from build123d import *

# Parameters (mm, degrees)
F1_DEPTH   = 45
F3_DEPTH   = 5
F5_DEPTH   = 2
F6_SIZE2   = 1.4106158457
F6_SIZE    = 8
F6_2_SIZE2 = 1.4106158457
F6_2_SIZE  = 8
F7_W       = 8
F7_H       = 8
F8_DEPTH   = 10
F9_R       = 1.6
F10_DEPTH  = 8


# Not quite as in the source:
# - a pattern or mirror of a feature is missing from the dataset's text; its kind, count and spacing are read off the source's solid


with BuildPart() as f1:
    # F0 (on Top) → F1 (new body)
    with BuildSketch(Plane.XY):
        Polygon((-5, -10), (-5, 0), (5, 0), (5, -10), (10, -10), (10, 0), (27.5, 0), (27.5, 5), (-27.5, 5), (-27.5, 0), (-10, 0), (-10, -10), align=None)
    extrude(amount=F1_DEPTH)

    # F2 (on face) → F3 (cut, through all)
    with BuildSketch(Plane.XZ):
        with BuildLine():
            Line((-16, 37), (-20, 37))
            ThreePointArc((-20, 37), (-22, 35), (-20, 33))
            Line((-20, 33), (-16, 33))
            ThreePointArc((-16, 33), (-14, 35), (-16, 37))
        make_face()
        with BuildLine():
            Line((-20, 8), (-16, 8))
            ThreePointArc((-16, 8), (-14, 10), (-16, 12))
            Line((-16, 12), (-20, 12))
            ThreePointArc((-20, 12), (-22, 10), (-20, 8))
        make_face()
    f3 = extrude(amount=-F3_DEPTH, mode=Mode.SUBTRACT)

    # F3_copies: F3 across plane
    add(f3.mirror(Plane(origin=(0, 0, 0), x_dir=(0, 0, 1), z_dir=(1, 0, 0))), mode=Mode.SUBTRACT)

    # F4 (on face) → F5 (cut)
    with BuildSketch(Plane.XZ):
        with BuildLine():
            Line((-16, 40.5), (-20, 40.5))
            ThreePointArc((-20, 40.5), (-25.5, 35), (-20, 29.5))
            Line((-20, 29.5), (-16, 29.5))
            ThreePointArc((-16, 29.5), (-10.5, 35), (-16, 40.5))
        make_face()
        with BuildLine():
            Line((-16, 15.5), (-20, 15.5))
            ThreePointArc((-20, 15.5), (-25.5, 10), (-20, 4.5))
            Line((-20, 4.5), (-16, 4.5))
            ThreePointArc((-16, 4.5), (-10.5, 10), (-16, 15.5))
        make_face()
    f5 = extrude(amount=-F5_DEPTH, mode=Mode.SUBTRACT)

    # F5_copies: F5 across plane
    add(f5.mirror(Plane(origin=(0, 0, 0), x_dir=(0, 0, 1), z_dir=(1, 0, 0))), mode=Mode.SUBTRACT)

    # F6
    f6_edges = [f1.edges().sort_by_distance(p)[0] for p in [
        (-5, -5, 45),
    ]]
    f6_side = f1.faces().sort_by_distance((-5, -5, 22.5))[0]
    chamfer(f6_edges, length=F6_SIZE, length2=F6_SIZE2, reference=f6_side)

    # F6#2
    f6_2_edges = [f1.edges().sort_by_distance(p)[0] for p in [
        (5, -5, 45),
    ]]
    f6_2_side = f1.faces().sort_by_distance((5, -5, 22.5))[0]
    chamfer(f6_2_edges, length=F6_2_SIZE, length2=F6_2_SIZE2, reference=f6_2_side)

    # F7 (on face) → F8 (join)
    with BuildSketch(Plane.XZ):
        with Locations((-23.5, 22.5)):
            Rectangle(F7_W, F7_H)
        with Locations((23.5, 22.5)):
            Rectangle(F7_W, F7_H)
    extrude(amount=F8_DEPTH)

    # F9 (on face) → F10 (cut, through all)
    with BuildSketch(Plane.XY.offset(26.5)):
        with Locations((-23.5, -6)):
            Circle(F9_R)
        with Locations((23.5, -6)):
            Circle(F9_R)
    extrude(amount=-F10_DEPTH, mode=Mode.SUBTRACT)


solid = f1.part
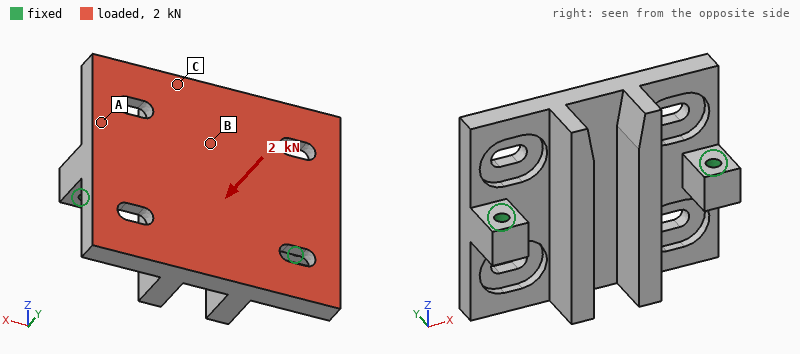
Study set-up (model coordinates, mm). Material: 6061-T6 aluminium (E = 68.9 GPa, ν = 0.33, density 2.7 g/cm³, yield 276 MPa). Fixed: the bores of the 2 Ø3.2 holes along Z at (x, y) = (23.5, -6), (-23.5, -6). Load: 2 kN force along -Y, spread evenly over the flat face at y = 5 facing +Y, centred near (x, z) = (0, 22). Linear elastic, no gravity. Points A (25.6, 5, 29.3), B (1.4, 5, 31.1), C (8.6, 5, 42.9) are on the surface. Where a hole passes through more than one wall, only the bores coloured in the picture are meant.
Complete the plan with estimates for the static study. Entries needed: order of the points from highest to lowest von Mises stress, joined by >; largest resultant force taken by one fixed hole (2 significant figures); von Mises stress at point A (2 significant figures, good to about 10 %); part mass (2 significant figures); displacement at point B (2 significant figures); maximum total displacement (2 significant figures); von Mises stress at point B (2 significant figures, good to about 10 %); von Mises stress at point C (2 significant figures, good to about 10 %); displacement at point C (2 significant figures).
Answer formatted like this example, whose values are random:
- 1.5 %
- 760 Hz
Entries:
- B > A > C
- 1.2 kN
- 20 MPa
- 44 g
- 32 µm
- 36 µm
- 27 MPa
- 5.6 MPa
- 32 µm
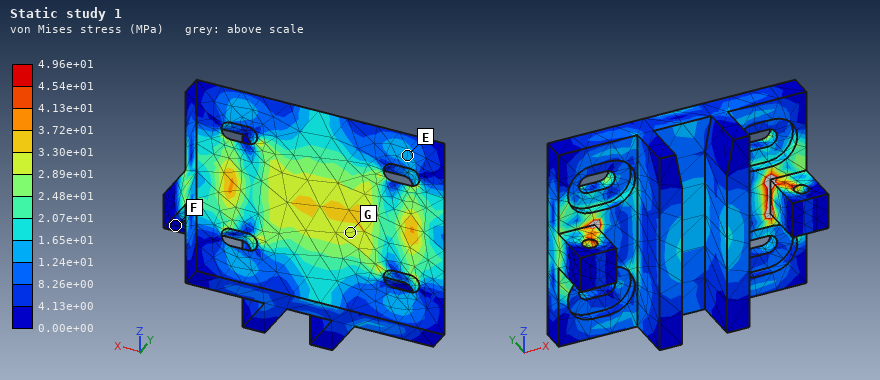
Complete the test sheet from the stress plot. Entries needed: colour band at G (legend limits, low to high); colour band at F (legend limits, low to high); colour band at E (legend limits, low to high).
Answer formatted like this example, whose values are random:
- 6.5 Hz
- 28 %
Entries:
- 2.89e+01 to 3.30e+01 MPa
- 0.00e+00 to 4.13e+00 MPa
- 1.24e+01 to 1.65e+01 MPa
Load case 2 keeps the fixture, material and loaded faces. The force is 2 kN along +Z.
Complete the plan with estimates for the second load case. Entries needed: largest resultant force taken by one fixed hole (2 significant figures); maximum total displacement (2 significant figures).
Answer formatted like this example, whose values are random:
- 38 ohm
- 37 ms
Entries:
- 1.0 kN
- 77 µm
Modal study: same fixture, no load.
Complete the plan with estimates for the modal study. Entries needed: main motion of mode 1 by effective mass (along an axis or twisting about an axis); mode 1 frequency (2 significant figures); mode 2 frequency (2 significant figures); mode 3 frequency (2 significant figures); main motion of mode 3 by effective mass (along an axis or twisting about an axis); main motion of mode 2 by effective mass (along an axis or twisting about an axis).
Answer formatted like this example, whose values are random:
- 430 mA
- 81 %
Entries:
- twisting about X
- 3200 Hz
- 6000 Hz
- 7900 Hz
- along X
- along Y
